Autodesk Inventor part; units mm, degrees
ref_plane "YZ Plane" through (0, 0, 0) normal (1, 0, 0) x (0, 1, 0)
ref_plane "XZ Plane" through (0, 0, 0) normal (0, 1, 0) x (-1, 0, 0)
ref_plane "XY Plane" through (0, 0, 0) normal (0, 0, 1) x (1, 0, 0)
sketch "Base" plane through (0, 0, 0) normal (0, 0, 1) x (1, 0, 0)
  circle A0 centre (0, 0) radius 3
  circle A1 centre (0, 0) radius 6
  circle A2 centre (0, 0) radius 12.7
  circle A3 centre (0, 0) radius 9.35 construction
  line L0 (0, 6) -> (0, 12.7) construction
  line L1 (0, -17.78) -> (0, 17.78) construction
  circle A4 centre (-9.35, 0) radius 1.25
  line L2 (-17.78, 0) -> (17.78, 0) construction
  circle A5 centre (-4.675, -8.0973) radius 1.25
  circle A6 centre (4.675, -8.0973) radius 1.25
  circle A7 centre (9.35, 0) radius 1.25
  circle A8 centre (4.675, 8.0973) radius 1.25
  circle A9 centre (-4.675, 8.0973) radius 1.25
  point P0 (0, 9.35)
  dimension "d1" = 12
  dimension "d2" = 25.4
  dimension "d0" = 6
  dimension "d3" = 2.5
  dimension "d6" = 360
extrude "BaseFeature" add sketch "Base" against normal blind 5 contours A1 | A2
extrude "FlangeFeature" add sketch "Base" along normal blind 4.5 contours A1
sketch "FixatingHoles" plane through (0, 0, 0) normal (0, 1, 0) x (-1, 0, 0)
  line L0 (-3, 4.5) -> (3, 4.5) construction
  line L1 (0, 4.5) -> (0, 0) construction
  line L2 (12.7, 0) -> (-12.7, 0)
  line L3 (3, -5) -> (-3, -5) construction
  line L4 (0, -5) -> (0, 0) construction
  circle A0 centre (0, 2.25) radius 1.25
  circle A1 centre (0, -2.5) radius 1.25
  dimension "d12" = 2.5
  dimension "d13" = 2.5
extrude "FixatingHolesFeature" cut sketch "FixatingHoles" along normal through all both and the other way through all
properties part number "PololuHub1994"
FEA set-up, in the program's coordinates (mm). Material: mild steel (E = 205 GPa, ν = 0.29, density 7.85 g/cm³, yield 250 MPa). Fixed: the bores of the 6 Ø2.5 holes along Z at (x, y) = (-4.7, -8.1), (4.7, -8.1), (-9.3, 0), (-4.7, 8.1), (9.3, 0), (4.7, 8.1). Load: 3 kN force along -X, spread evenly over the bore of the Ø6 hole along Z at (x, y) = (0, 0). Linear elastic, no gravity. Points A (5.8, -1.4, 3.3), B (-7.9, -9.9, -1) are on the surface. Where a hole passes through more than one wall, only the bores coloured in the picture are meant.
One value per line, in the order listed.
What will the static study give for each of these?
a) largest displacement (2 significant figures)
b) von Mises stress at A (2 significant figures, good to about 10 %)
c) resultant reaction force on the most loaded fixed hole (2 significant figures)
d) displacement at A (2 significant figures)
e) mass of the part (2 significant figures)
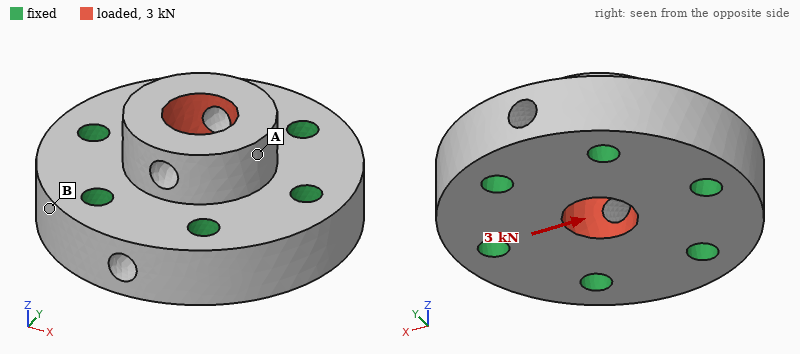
2.9 µm
20 MPa
860 N
2.3 µm
20 g
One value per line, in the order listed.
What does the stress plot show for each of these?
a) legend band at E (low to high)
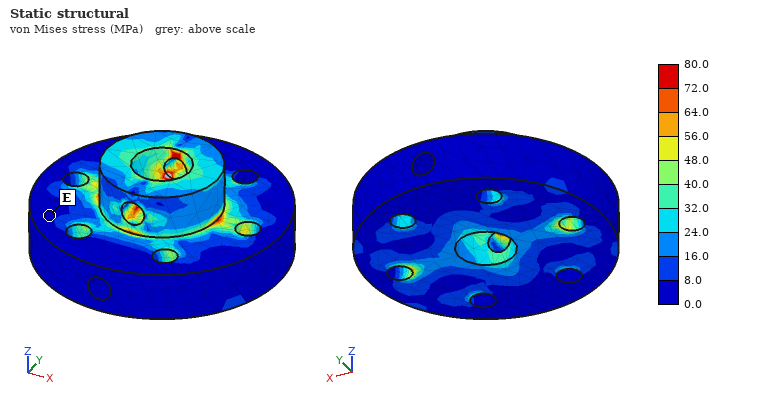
0.0 to 8.0 MPa
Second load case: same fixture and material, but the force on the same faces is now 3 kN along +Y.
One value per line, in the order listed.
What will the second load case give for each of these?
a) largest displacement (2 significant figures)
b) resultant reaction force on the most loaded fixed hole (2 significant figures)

2.5 µm
690 N
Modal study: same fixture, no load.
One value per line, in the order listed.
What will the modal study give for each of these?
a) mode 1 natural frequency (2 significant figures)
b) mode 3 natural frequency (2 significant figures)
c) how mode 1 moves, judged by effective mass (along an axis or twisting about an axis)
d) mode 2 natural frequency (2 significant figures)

86 kHz
90 kHz
along X
89 kHz
